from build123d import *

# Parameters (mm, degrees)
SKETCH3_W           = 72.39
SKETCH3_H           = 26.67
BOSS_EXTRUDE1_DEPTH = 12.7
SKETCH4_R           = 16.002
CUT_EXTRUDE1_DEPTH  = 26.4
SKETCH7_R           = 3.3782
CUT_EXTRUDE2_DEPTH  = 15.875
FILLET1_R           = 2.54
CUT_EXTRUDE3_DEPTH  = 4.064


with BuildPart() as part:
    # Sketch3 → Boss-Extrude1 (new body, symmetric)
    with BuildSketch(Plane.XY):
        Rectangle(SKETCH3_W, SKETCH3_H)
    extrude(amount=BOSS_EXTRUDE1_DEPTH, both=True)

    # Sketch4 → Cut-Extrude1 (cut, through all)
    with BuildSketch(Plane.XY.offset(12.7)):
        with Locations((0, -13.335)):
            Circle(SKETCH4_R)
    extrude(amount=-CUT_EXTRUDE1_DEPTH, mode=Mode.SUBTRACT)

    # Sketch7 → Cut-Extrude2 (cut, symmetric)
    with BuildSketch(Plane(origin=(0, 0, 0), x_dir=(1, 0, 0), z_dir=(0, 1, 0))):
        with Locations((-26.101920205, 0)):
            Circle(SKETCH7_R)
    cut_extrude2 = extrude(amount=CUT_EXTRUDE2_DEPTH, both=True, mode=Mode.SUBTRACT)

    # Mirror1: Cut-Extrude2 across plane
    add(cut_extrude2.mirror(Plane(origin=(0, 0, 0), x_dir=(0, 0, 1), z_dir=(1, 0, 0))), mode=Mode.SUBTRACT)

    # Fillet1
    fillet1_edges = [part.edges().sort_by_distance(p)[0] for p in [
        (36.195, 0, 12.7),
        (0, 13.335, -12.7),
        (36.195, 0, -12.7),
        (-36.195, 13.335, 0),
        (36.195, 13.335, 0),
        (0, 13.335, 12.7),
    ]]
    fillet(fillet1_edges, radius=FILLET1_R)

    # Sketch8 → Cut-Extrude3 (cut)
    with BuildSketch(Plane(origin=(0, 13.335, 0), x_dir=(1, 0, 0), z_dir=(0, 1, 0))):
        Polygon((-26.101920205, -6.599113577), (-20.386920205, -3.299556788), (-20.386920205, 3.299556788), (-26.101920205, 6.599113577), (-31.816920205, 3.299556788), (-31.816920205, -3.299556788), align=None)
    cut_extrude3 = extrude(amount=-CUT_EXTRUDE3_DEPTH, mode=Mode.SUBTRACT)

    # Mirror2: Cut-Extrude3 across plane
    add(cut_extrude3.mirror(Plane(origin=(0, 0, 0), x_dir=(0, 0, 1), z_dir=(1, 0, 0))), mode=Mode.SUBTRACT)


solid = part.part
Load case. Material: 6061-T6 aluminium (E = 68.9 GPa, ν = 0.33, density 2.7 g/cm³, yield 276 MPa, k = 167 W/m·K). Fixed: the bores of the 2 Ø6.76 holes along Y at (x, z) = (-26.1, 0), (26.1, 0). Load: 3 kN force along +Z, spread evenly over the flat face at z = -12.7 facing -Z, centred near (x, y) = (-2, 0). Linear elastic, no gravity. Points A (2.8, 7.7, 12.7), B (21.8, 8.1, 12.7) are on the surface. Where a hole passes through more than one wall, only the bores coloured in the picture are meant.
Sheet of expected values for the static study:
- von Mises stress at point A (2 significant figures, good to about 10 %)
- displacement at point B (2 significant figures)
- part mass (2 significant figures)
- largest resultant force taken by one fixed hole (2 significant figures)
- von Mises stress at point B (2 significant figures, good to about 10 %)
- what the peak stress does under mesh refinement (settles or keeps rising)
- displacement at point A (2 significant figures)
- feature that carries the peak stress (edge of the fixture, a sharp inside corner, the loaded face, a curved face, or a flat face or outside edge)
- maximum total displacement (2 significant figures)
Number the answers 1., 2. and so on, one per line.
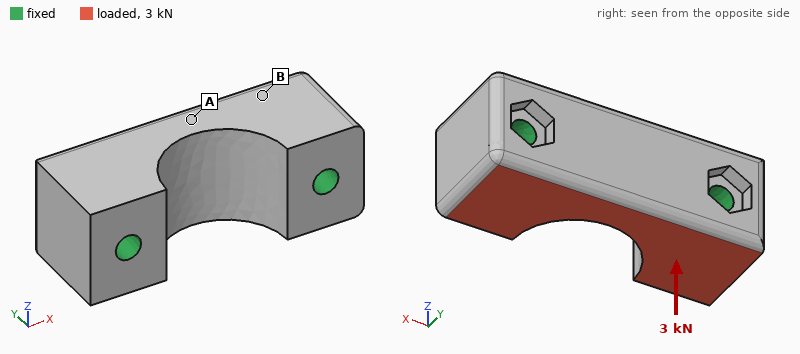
1. 3.4 MPa
2. 0.85 µm
3. 97 g
4. 1.6 kN
5. 1.0 MPa
6. keeps rising
7. 1.7 µm
8. edge of the fixture
9. 2.2 µm
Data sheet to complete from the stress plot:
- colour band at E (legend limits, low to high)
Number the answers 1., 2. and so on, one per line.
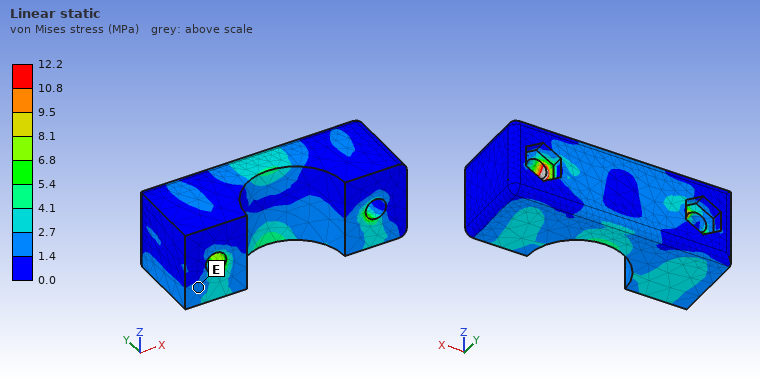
1. 1.4 to 2.7 MPa
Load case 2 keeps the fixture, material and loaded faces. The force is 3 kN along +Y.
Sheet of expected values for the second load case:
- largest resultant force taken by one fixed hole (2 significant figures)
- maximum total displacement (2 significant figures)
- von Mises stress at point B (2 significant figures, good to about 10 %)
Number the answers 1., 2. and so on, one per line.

1. 1.6 kN
2. 4.8 µm
3. 2.0 MPa
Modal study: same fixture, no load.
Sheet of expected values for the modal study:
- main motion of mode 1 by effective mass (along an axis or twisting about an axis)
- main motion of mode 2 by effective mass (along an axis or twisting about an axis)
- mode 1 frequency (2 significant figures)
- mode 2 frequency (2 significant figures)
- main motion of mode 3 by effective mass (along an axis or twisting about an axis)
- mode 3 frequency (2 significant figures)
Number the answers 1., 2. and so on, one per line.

1. along Z
2. along Y
3. 20 kHz
4. 26 kHz
5. twisting about X
6. 33 kHz
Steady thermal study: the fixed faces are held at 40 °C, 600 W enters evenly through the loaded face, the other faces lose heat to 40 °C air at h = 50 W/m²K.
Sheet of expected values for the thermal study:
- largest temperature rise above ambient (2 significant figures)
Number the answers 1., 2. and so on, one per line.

1. 52 K
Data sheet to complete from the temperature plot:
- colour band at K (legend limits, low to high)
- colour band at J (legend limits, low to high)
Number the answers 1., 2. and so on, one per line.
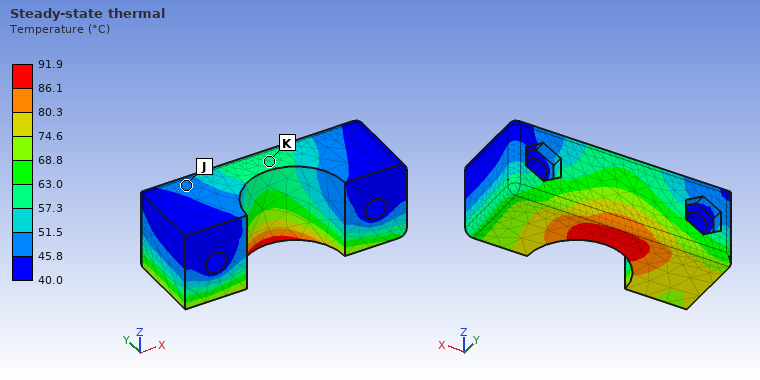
1. 57.3 to 63.0 °C
2. 45.8 to 51.5 °C
